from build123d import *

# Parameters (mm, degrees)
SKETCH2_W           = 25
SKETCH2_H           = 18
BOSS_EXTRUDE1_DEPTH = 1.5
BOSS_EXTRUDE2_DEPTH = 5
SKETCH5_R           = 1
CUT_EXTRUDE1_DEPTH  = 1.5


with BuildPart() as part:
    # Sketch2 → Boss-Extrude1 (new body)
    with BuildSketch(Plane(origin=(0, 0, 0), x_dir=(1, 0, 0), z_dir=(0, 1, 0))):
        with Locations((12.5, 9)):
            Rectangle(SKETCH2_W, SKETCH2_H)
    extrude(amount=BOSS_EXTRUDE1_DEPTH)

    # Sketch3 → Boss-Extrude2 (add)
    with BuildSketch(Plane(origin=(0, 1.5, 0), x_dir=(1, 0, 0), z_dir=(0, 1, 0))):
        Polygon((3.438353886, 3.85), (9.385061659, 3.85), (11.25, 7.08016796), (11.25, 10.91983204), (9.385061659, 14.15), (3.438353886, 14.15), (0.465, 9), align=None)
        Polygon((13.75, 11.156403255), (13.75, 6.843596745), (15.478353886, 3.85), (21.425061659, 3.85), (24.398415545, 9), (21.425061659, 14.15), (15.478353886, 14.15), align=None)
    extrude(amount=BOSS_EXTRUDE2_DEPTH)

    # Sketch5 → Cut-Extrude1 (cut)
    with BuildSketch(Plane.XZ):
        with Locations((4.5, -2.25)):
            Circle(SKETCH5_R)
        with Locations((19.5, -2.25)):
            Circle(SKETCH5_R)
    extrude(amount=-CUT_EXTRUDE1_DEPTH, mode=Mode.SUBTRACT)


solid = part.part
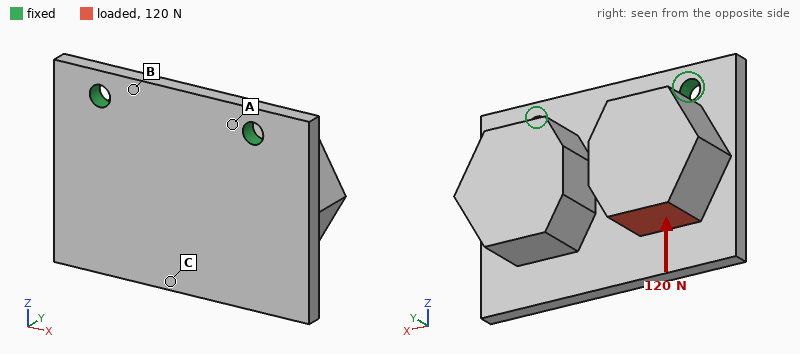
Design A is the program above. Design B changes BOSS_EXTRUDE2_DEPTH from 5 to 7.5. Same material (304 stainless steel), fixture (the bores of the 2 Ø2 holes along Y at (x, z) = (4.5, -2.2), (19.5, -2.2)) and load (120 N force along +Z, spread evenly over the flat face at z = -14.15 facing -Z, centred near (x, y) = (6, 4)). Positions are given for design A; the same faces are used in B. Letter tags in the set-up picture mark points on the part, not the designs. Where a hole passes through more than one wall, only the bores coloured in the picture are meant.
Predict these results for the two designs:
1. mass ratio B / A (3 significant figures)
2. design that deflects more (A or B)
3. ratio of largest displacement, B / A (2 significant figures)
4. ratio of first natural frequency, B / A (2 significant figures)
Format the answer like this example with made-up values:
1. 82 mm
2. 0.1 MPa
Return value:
1. 1.29
2. B
3. 1.4
4. 0.83
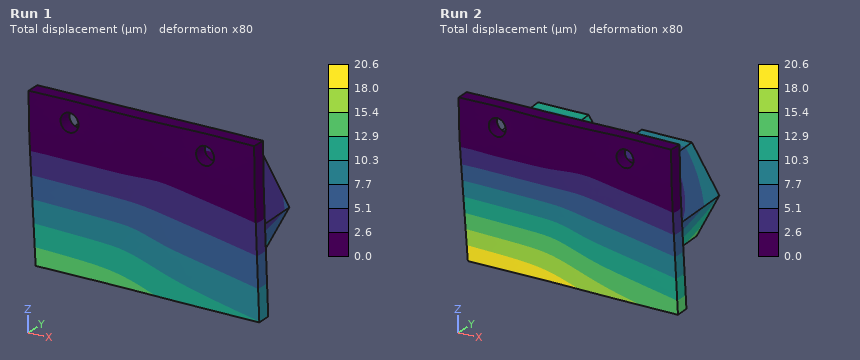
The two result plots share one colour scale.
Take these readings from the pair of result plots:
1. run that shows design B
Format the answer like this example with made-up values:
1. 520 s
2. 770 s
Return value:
1. Run 2
